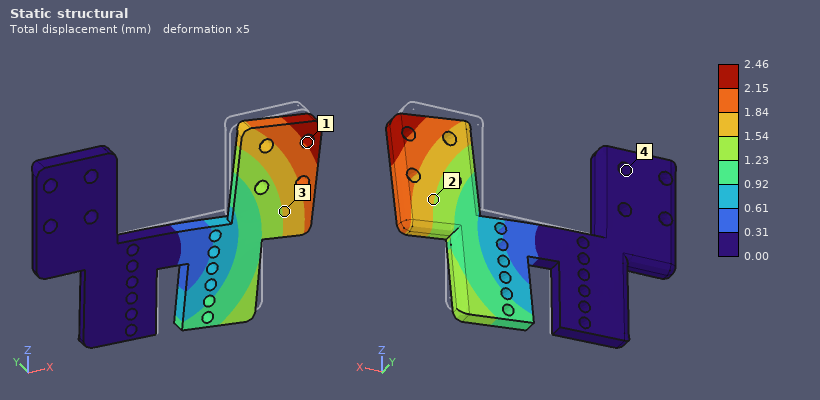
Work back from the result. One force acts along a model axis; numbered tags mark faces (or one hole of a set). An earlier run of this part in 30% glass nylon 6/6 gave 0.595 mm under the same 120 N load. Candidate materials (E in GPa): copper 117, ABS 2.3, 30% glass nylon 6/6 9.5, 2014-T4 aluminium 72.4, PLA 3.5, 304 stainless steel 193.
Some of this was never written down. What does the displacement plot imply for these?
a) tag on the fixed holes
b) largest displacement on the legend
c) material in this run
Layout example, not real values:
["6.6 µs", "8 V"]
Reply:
["4", "2.46 mm", "ABS"]
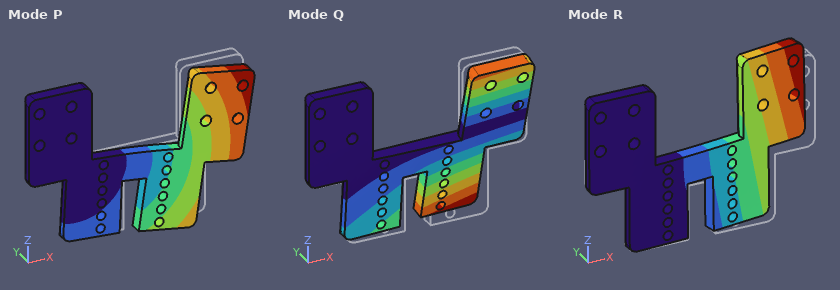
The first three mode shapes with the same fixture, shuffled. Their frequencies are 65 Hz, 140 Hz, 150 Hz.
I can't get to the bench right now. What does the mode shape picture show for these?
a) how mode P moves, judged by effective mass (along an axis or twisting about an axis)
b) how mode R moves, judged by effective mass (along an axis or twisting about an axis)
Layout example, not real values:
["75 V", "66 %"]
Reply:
["along Z", "along Y"]
